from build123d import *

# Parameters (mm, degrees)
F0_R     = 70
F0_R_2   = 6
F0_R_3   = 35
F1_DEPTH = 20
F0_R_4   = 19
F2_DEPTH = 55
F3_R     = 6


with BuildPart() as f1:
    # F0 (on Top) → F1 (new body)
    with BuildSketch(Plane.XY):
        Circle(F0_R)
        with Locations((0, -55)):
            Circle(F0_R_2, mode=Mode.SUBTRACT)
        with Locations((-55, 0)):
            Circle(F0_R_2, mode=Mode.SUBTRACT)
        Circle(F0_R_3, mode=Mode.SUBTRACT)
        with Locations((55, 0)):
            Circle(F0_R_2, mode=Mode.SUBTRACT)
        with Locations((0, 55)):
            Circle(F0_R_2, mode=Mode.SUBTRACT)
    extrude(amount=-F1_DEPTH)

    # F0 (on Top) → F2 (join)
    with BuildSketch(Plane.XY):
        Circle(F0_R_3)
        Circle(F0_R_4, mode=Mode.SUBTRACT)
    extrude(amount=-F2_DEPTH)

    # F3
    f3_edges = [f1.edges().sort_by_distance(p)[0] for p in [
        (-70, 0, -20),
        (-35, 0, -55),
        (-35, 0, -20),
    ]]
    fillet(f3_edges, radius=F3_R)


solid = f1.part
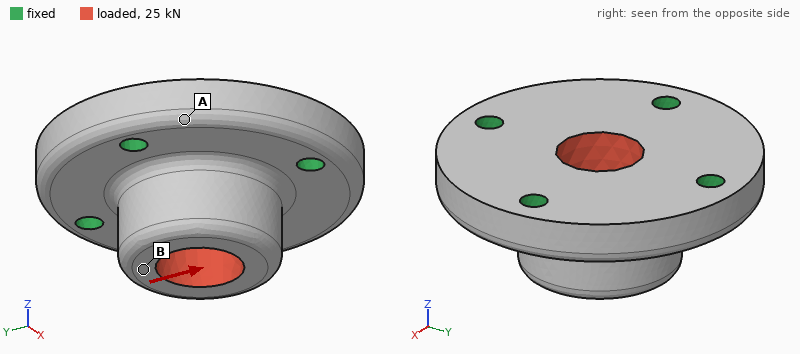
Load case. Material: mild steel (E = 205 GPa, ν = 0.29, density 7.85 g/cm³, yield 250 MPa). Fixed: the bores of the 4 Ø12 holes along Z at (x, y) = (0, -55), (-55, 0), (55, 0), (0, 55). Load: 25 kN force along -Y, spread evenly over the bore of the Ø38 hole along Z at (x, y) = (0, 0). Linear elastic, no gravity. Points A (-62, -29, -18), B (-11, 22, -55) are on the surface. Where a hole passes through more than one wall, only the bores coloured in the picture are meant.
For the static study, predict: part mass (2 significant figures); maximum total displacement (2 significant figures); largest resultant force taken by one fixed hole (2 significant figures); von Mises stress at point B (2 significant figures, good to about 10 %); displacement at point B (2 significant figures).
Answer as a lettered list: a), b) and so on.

a) 2.9 kg
b) 6.6 µm
c) 8.8 kN
d) 8.2 MPa
e) 6.4 µm
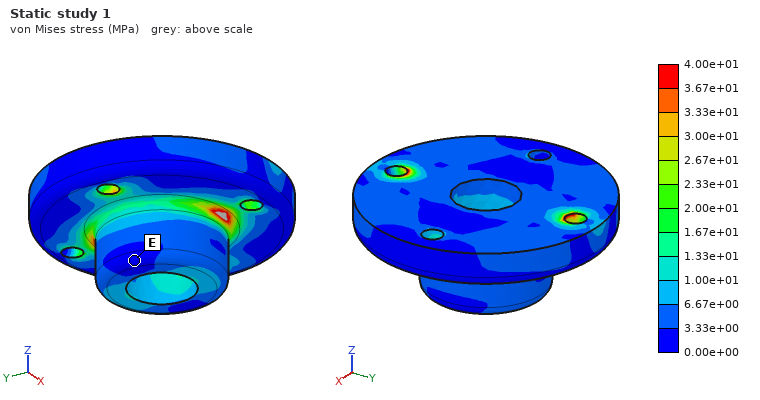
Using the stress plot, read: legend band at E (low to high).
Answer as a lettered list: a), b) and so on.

a) 0.00e+00 to 3.33e+00 MPa
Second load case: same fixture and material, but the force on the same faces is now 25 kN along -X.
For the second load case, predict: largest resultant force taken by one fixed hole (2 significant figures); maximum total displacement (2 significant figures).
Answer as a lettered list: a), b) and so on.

a) 8.8 kN
b) 6.6 µm
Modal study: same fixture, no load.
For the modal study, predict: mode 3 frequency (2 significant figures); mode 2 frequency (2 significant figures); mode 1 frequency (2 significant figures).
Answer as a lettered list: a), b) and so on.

a) 9600 Hz
b) 9500 Hz
c) 9500 Hz
